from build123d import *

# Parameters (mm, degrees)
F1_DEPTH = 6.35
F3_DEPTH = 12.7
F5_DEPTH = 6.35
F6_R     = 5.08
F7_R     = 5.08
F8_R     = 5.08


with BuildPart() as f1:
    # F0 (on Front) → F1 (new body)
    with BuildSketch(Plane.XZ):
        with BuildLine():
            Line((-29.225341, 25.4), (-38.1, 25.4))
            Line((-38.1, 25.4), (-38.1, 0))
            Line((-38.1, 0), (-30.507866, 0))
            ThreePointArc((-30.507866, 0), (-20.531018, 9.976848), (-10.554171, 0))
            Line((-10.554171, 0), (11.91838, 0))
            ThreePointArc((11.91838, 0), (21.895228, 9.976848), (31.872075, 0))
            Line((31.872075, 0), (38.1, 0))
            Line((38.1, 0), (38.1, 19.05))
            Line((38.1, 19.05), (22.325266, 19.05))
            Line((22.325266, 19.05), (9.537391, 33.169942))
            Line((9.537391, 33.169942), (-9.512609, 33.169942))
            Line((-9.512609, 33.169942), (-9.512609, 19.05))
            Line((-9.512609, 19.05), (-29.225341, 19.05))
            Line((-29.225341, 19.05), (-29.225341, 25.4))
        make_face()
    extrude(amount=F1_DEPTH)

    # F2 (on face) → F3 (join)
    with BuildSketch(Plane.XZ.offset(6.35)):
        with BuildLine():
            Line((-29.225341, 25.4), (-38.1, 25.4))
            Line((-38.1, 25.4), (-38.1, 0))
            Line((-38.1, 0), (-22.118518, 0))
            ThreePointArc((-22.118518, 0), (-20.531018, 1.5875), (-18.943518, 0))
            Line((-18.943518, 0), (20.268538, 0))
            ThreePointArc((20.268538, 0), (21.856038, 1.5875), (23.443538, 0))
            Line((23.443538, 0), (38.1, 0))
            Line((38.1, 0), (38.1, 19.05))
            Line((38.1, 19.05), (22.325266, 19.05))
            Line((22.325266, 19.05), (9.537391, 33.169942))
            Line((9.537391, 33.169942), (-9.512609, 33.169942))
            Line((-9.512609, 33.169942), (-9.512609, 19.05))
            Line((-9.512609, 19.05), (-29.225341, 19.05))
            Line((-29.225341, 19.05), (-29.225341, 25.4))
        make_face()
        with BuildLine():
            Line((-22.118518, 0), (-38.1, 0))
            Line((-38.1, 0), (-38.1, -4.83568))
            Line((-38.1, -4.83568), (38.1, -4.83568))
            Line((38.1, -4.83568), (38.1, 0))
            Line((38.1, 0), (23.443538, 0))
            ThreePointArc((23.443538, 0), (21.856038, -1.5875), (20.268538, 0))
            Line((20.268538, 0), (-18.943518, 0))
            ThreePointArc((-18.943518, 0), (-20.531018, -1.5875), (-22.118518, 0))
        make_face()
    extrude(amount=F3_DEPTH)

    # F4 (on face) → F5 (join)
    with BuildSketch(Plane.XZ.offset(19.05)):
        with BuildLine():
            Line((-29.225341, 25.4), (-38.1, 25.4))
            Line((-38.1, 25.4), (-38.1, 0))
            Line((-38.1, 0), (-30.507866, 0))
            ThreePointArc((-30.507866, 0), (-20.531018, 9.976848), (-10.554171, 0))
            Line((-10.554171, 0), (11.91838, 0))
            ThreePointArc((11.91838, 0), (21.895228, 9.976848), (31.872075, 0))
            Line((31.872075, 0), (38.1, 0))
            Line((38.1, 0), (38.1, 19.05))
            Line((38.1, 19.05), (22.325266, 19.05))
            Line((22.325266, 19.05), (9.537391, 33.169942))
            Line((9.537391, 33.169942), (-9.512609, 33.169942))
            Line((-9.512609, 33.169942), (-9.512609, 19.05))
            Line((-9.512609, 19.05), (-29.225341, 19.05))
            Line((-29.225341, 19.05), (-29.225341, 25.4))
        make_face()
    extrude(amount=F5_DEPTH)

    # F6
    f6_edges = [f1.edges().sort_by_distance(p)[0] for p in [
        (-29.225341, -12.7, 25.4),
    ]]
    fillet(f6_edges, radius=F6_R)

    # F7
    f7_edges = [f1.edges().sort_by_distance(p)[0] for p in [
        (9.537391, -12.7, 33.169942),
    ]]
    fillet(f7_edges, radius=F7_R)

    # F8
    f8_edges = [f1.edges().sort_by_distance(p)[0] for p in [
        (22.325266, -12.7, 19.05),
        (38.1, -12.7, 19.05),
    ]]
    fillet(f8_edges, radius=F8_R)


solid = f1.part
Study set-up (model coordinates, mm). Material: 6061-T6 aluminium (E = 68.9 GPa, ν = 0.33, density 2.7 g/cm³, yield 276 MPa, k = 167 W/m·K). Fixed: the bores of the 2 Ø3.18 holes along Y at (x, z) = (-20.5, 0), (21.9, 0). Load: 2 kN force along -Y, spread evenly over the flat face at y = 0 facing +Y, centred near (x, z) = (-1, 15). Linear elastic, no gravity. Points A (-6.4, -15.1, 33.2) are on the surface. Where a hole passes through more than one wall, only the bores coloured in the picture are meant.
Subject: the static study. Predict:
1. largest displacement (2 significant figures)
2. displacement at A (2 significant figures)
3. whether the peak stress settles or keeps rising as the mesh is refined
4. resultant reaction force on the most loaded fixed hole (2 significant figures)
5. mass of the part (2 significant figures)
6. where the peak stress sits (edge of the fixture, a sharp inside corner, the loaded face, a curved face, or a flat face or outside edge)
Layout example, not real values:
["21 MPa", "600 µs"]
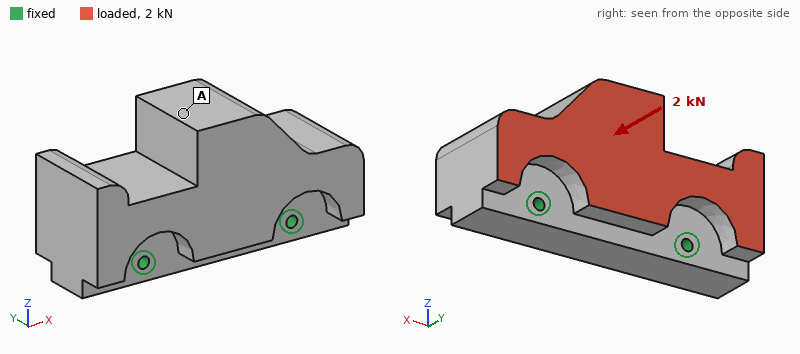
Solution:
["25 µm", "23 µm", "keeps rising", "1.0 kN", "130 g", "edge of the fixture"]
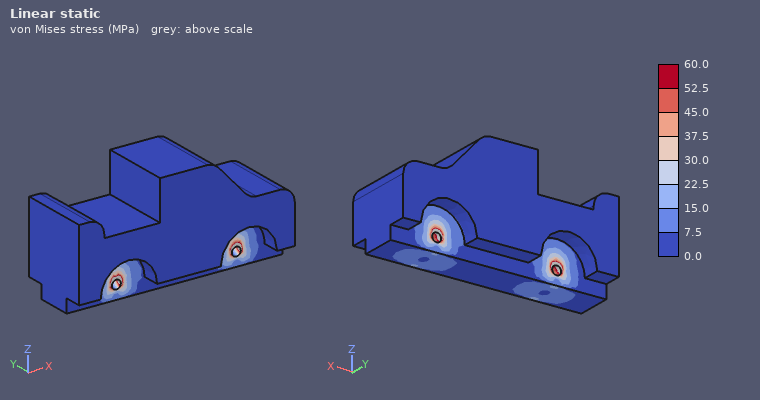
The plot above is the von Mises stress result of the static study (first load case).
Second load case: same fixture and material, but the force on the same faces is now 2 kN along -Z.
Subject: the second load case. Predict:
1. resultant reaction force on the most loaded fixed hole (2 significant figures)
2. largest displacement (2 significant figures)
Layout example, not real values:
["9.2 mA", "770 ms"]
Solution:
["1.1 kN", "24 µm"]
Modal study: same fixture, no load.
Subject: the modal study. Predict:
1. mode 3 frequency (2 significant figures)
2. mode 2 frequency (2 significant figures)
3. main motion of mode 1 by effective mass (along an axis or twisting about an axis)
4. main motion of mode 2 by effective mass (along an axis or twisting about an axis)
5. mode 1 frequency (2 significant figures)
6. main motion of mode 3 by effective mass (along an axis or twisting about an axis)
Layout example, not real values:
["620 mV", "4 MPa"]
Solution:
["13 kHz", "11 kHz", "along Y", "twisting about Z", "5500 Hz", "along X"]
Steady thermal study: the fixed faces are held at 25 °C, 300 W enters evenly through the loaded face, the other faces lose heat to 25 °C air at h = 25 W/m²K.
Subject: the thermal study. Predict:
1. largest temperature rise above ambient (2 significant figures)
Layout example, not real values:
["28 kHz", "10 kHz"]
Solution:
["57 K"]
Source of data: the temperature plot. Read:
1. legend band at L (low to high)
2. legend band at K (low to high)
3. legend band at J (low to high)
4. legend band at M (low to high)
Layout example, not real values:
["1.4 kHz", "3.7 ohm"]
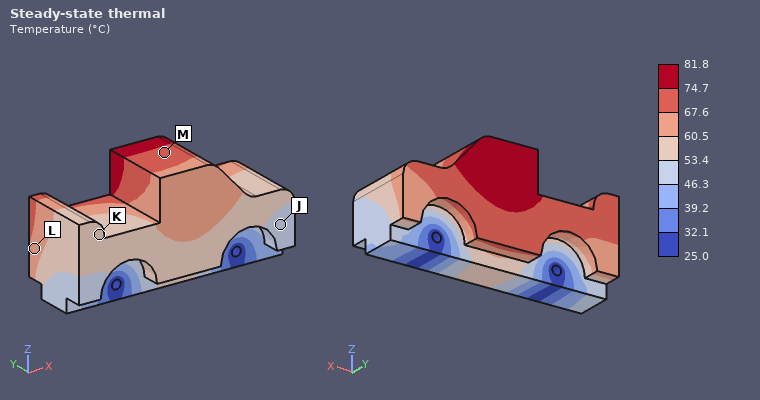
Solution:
["60.5 to 67.6 °C", "53.4 to 60.5 °C", "46.3 to 53.4 °C", "67.6 to 74.7 °C"]
